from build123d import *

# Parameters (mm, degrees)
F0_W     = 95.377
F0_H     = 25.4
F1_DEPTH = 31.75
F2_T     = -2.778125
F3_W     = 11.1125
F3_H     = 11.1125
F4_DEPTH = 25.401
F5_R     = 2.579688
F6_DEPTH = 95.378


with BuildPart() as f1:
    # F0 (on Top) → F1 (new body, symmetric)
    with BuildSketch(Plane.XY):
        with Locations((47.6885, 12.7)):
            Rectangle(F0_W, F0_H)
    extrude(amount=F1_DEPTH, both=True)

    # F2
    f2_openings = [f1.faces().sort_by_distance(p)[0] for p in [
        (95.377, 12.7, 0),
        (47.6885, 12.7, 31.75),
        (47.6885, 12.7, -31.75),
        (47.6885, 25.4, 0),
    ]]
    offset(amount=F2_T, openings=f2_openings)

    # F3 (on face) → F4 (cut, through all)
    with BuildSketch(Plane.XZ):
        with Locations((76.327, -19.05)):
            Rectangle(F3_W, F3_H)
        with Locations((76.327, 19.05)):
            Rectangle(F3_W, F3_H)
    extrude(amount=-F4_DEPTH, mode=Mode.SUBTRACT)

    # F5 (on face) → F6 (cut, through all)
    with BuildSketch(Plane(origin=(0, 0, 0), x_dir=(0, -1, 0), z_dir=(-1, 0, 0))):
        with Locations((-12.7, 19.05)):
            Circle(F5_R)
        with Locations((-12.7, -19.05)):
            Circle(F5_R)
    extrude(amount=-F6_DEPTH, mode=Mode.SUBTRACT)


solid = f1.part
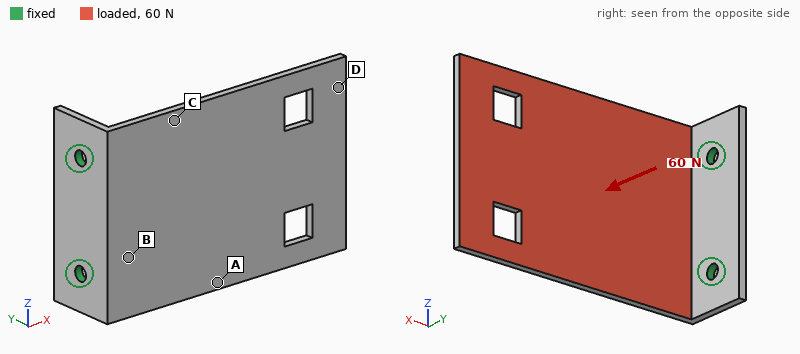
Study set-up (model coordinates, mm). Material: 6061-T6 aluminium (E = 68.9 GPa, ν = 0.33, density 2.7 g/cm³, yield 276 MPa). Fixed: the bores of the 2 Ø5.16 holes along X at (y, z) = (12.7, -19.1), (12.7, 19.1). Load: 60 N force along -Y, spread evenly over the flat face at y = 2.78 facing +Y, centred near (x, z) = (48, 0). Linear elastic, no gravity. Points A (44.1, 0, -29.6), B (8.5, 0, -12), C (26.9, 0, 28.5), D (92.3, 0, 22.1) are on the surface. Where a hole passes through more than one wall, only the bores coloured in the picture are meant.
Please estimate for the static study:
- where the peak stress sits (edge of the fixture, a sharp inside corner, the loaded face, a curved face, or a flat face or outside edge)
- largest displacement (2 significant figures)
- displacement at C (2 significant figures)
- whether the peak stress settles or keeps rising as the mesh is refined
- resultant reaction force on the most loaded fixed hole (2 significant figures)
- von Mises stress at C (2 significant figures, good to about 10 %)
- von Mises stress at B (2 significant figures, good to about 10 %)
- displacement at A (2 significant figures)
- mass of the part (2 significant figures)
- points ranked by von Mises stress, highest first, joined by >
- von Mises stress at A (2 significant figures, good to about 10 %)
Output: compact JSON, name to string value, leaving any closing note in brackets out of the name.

{"where the peak stress sits": "edge of the fixture", "largest displacement": "1.1 mm", "displacement at C": "0.18 mm", "whether the peak stress settles or keeps rising as the mesh is refined": "keeps rising", "resultant reaction force on the most loaded fixed hole": "31 N", "von Mises stress at C": "18 MPa", "von Mises stress at B": "27 MPa", "displacement at A": "0.36 mm", "mass of the part": "54 g", "points ranked by von Mises stress, highest first, joined by >": "B > C > A > D", "von Mises stress at A": "10 MPa"}
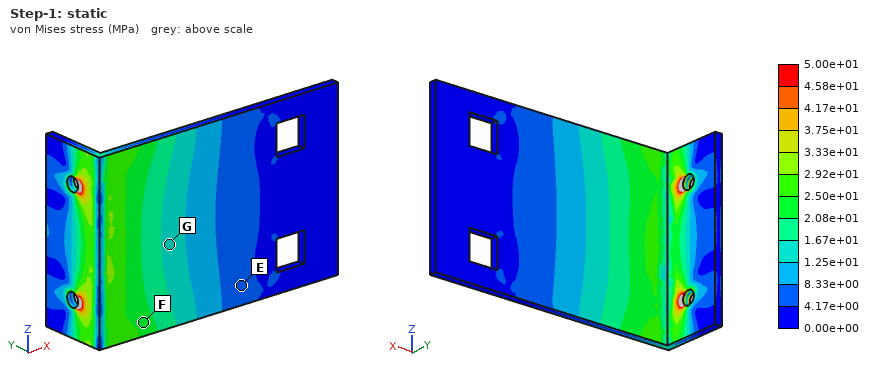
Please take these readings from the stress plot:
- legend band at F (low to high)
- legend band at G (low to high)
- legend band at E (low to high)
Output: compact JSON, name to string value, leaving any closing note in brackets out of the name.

{"legend band at F": "2.08e+01 to 2.50e+01 MPa", "legend band at G": "1.25e+01 to 1.67e+01 MPa", "legend band at E": "4.17e+00 to 8.33e+00 MPa"}
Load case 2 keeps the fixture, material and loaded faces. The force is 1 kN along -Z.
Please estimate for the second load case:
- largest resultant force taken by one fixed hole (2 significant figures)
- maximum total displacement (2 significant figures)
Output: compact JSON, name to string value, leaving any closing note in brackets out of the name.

{"largest resultant force taken by one fixed hole": "1.3 kN", "maximum total displacement": "0.73 mm"}
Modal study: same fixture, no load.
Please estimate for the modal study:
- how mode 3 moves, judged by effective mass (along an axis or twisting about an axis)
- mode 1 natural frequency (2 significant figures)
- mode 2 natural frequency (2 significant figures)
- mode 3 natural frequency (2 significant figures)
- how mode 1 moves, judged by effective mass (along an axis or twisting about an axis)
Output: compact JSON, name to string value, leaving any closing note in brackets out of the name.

{"how mode 3 moves, judged by effective mass": "along Z", "mode 1 natural frequency": "230 Hz", "mode 2 natural frequency": "810 Hz", "mode 3 natural frequency": "1300 Hz", "how mode 1 moves, judged by effective mass": "along Y"}
